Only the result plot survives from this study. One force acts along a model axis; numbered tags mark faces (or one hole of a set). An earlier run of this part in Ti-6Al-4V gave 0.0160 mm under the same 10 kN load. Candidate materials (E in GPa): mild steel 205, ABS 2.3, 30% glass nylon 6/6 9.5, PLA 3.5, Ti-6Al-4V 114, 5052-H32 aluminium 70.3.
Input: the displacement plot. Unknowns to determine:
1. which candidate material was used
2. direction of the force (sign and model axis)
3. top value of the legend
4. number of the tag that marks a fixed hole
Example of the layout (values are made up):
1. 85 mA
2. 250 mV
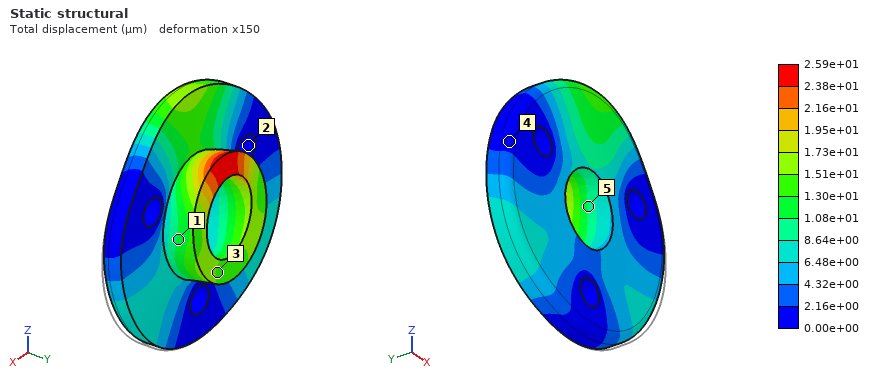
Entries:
1. 5052-H32 aluminium
2. +Z
3. 2.59e+01 µm
4. 2
